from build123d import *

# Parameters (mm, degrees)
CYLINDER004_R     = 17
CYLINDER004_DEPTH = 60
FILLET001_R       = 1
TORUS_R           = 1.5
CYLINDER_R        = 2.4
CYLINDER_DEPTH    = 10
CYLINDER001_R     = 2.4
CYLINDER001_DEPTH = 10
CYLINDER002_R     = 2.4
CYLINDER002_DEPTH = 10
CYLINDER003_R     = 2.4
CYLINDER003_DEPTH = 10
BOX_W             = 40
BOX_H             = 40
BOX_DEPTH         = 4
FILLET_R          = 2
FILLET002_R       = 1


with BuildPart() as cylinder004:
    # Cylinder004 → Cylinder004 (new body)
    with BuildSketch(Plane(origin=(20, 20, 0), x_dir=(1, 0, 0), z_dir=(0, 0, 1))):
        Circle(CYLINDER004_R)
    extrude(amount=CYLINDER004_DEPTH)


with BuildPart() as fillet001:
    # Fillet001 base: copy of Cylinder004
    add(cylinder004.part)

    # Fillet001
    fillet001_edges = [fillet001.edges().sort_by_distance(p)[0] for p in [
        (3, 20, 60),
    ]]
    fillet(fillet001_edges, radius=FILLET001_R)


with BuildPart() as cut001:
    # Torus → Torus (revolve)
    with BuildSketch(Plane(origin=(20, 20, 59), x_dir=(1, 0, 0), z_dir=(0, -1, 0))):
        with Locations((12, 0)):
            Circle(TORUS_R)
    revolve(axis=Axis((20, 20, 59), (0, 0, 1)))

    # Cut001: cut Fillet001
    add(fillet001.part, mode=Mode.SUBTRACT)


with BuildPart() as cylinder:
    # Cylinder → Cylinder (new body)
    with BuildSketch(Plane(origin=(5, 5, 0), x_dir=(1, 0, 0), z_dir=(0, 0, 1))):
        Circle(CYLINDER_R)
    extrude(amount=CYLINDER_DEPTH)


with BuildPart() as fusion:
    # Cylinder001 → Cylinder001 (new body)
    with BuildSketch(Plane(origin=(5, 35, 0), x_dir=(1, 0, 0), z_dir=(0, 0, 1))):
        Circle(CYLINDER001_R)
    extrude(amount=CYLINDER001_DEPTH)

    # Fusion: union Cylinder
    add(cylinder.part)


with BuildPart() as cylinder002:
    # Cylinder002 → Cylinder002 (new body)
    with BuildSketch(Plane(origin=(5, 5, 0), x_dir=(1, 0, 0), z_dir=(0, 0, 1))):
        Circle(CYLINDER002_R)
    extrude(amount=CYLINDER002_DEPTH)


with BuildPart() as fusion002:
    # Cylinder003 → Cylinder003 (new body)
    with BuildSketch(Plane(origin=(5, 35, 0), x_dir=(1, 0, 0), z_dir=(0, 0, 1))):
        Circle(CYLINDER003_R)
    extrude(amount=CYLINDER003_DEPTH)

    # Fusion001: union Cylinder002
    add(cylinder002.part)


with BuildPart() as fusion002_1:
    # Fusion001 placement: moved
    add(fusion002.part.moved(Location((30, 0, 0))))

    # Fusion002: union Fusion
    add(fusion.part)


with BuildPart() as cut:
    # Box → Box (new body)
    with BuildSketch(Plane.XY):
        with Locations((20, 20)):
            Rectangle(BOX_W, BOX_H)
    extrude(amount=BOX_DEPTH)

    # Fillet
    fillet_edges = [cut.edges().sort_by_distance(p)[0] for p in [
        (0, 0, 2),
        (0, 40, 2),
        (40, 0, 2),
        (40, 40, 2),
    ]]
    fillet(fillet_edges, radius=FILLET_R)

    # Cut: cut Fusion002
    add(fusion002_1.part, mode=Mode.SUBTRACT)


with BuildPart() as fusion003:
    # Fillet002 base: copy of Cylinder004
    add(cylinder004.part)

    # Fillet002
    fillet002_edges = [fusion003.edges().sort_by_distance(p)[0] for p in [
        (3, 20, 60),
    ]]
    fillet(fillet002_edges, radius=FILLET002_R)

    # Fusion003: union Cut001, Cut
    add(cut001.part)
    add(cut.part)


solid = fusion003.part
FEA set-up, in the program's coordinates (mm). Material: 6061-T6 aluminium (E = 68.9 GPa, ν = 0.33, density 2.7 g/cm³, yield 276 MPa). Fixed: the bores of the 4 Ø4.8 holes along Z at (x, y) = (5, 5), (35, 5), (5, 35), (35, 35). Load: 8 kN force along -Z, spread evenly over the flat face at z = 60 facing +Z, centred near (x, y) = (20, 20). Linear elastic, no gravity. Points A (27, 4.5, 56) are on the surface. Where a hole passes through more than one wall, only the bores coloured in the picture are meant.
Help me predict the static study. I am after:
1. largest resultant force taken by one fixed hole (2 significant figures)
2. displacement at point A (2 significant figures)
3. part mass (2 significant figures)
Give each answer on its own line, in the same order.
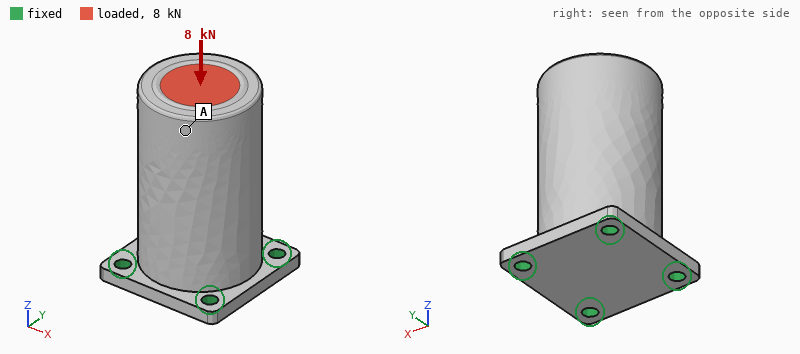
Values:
2.2 kN
19 µm
150 g
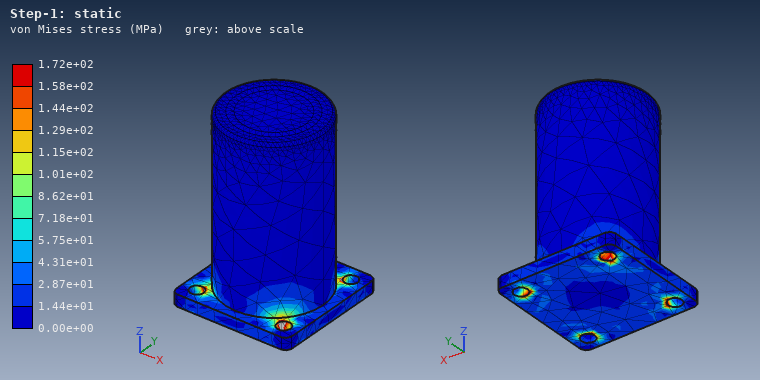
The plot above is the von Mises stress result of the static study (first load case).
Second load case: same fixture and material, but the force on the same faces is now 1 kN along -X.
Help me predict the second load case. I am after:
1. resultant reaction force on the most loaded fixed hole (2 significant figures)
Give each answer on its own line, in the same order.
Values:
1.2 kN
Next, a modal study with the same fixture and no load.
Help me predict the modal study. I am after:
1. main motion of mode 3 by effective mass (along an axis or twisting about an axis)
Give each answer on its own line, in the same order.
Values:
along Z
